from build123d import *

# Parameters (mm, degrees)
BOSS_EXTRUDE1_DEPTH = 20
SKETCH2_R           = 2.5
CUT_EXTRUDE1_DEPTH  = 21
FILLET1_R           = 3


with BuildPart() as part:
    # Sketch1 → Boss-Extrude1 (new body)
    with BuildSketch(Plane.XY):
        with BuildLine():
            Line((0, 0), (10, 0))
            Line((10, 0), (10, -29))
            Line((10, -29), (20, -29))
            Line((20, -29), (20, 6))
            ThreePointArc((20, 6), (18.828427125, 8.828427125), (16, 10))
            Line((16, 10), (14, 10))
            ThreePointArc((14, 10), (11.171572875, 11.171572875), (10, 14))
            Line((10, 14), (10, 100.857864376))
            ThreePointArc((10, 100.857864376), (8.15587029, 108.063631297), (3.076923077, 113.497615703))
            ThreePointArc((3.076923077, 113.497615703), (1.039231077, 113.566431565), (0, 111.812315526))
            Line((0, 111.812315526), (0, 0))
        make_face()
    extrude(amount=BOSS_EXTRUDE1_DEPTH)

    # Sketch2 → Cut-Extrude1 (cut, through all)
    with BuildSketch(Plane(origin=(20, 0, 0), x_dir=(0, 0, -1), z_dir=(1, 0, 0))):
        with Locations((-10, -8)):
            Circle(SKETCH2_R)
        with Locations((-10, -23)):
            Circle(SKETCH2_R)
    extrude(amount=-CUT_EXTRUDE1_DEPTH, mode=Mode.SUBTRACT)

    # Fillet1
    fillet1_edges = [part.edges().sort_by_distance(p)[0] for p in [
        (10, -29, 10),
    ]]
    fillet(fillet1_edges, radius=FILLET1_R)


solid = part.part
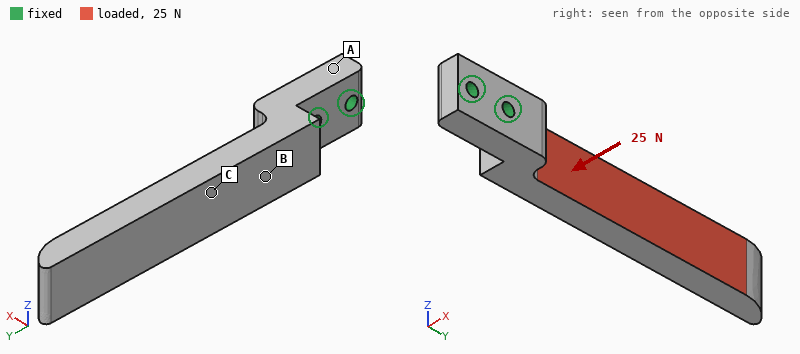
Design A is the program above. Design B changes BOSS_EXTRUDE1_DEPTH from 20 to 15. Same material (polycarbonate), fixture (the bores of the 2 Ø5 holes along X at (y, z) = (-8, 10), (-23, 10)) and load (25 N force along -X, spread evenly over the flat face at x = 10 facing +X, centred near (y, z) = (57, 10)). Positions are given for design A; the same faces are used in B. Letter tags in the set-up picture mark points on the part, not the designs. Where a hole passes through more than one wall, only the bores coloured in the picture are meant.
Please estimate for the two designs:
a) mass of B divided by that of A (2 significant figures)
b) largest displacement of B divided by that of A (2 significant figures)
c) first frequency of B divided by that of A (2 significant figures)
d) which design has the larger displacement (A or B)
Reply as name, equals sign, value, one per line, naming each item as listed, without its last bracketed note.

mass of B divided by that of A = 0.75
largest displacement of B divided by that of A = 1.3
first frequency of B divided by that of A = 1.0
which design has the larger displacement = B
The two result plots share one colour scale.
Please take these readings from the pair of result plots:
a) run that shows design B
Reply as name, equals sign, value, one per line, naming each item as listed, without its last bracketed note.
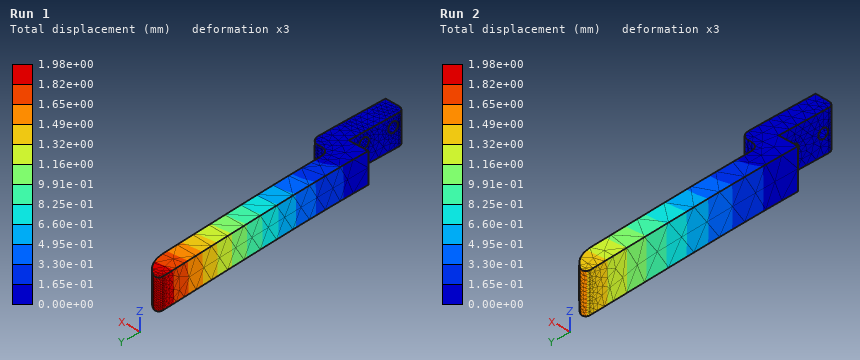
run that shows design B = Run 1
